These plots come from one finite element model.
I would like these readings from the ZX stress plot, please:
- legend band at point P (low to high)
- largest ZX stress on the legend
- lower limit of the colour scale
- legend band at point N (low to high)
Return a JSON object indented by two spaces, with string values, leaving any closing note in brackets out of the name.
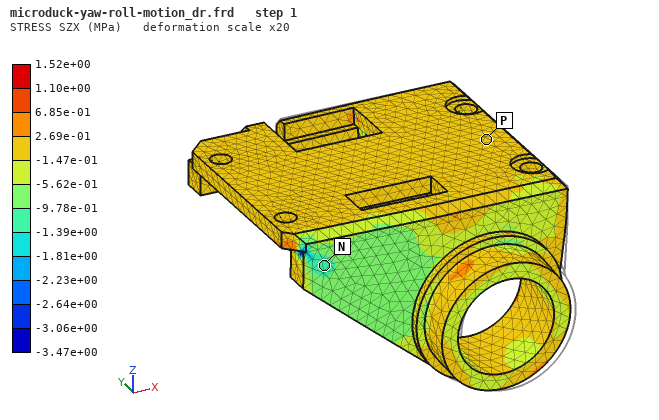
{
  "legend band at point P": "-1.47e-01 to 2.69e-01 MPa",
  "largest ZX stress on the legend": "1.52e+00 MPa",
  "lower limit of the colour scale": "-3.47e+00 MPa",
  "legend band at point N": "-1.39e+00 to -9.78e-01 MPa"
}
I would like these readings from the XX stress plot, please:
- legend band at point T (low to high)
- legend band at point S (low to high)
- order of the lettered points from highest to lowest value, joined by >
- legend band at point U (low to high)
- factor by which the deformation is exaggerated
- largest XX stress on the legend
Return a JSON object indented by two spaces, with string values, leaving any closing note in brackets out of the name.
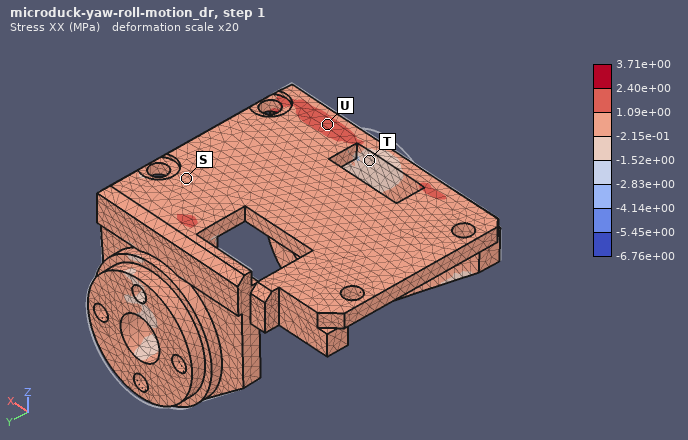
{
  "legend band at point T": "-1.52e+00 to -2.15e-01 MPa",
  "legend band at point S": "-2.15e-01 to 1.09e+00 MPa",
  "order of the lettered points from highest to lowest value, joined by >": "U > S > T",
  "legend band at point U": "1.09e+00 to 2.40e+00 MPa",
  "factor by which the deformation is exaggerated": "20",
  "largest XX stress on the legend": "3.71e+00 MPa"
}
